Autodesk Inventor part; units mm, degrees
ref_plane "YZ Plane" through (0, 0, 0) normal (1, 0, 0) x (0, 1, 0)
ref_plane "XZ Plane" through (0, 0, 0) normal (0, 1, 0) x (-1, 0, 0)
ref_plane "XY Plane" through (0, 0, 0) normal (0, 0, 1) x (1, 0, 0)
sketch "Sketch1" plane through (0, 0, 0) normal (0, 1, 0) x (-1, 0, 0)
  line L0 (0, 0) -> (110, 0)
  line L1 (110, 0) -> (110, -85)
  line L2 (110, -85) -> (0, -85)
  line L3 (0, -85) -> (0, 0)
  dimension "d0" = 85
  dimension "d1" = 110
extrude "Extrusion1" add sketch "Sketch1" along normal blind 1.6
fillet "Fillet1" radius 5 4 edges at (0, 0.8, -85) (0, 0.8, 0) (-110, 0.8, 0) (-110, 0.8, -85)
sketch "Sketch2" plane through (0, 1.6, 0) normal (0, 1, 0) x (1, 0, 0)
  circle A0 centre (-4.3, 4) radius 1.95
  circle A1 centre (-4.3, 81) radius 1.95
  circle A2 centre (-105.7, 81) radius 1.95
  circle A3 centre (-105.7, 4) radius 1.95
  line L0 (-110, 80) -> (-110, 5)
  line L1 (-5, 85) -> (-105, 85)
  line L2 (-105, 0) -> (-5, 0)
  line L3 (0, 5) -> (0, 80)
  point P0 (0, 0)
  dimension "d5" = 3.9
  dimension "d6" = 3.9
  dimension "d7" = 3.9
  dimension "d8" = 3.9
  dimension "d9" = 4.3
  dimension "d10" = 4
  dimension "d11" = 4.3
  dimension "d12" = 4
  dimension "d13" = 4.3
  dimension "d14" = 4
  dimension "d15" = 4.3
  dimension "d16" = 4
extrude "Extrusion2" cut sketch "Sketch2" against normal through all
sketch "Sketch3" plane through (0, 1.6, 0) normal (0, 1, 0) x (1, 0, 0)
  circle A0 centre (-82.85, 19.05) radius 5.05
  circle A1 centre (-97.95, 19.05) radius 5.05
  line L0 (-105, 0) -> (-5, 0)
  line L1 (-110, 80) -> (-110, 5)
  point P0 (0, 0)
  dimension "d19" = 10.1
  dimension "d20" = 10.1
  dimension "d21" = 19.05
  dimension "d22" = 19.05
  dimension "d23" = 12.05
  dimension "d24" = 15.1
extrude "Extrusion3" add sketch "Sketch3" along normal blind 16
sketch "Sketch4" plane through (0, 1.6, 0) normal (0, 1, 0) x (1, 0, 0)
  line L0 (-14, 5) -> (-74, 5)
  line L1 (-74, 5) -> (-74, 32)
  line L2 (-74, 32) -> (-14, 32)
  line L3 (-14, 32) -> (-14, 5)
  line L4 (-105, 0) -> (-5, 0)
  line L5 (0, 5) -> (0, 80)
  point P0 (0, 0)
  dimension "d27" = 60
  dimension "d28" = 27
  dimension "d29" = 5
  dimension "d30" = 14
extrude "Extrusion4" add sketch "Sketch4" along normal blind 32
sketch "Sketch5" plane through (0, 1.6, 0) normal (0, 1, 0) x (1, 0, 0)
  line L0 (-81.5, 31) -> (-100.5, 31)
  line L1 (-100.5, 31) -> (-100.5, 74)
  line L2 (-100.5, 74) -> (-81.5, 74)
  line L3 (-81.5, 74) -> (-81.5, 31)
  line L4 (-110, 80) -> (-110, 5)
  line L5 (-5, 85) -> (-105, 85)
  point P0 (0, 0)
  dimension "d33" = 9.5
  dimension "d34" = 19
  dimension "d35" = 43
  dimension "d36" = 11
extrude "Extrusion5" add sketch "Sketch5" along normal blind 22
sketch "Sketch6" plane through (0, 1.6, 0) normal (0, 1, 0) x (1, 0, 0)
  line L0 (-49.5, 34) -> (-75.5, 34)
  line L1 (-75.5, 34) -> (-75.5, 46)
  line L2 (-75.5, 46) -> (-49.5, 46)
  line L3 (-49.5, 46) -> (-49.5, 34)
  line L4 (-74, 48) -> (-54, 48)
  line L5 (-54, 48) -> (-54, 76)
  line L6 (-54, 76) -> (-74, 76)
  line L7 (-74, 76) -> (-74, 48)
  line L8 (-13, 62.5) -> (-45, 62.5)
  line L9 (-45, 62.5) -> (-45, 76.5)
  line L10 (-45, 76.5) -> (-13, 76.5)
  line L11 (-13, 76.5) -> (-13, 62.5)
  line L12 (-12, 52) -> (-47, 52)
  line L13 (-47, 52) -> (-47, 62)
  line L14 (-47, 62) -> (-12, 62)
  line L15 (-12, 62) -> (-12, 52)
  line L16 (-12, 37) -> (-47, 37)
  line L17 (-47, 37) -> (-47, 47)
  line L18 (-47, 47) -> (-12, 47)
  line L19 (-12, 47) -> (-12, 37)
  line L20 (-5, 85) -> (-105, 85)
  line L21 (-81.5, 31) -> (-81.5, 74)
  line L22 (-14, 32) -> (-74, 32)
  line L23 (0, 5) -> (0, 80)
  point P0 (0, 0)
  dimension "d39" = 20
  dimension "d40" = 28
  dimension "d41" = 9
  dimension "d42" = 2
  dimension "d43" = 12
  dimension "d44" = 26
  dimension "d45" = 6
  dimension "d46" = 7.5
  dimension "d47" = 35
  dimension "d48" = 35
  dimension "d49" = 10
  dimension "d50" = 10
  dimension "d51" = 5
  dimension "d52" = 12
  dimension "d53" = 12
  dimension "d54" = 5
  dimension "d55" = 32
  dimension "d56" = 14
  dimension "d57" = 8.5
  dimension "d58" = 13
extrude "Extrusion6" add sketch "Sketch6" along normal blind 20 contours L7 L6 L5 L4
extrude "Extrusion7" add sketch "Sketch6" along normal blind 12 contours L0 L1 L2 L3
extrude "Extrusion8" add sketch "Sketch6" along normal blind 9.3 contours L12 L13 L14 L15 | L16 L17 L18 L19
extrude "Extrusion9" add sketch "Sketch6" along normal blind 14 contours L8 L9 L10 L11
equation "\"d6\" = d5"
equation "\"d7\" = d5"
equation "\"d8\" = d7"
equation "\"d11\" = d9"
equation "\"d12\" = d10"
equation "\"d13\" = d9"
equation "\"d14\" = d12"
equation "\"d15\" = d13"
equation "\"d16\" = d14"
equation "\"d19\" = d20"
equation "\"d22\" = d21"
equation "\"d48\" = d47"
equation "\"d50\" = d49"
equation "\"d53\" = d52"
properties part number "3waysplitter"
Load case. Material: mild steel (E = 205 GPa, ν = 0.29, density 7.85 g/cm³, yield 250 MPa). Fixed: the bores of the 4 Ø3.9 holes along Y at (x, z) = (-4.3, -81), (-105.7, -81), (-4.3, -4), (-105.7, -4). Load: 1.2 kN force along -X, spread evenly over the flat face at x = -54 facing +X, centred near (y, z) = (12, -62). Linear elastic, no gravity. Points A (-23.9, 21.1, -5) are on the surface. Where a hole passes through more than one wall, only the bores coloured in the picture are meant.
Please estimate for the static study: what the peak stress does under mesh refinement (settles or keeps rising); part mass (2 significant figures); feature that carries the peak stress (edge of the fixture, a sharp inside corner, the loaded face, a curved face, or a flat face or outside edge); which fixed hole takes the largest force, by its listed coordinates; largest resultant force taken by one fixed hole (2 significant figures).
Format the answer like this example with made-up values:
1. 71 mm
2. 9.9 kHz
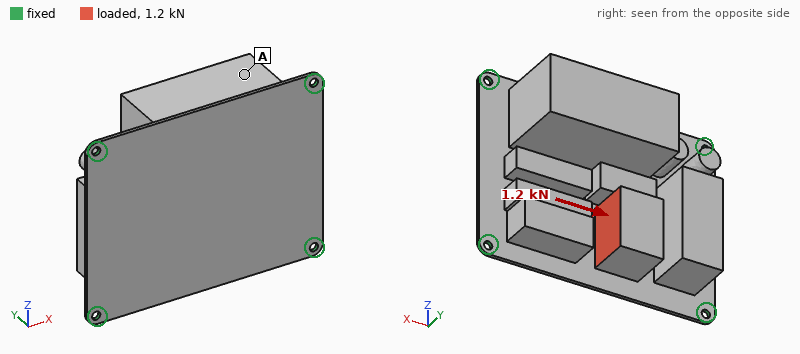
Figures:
1. keeps rising
2. 900 g
3. edge of the fixture
4. (-105.7, -81)
5. 410 N
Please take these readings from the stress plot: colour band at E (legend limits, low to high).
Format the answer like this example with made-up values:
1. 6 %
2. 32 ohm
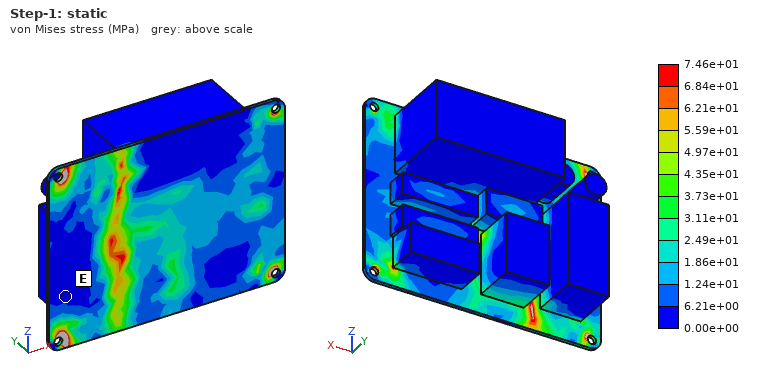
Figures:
1. 0.00e+00 to 6.21e+00 MPa
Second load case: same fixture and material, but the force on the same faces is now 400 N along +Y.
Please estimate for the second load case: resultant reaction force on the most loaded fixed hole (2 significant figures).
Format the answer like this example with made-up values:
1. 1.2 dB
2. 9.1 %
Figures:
1. 180 N
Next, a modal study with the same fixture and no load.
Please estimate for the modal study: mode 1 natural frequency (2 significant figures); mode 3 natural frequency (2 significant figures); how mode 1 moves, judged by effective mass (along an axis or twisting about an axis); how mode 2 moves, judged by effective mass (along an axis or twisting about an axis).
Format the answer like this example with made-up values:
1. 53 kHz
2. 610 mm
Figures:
1. 400 Hz
2. 1000 Hz
3. along Y
4. along Z
